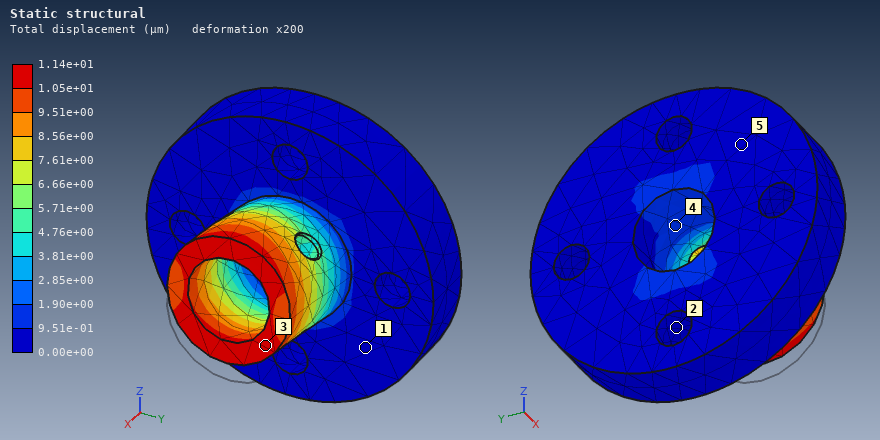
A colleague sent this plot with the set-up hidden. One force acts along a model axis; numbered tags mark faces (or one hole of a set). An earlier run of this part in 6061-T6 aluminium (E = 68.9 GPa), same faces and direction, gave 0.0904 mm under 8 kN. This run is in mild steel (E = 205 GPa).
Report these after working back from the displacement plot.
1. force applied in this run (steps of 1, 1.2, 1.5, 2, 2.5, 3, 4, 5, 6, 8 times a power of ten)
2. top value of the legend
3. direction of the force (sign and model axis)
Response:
3 kN
1.14e+01 µm
+Z
